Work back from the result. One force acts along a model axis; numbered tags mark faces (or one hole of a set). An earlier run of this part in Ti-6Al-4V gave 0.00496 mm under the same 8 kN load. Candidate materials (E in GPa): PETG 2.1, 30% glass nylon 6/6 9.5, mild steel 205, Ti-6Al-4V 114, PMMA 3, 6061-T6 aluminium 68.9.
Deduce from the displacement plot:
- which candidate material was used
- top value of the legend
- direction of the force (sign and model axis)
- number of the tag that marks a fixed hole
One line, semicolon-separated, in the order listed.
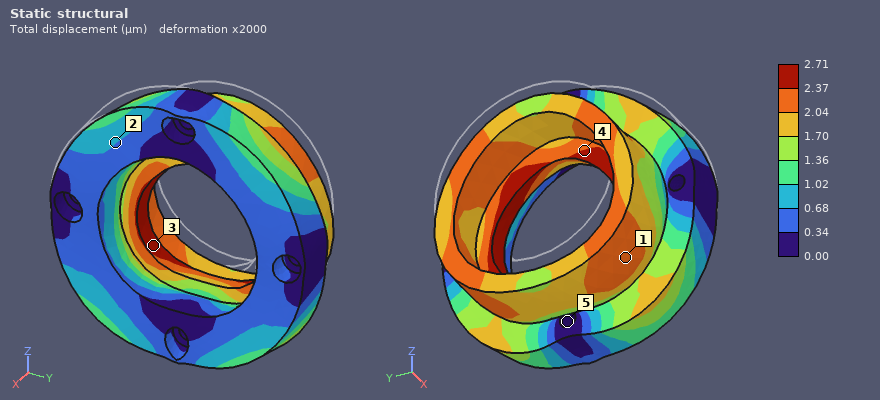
mild steel; 2.71 µm; -Z; 5
